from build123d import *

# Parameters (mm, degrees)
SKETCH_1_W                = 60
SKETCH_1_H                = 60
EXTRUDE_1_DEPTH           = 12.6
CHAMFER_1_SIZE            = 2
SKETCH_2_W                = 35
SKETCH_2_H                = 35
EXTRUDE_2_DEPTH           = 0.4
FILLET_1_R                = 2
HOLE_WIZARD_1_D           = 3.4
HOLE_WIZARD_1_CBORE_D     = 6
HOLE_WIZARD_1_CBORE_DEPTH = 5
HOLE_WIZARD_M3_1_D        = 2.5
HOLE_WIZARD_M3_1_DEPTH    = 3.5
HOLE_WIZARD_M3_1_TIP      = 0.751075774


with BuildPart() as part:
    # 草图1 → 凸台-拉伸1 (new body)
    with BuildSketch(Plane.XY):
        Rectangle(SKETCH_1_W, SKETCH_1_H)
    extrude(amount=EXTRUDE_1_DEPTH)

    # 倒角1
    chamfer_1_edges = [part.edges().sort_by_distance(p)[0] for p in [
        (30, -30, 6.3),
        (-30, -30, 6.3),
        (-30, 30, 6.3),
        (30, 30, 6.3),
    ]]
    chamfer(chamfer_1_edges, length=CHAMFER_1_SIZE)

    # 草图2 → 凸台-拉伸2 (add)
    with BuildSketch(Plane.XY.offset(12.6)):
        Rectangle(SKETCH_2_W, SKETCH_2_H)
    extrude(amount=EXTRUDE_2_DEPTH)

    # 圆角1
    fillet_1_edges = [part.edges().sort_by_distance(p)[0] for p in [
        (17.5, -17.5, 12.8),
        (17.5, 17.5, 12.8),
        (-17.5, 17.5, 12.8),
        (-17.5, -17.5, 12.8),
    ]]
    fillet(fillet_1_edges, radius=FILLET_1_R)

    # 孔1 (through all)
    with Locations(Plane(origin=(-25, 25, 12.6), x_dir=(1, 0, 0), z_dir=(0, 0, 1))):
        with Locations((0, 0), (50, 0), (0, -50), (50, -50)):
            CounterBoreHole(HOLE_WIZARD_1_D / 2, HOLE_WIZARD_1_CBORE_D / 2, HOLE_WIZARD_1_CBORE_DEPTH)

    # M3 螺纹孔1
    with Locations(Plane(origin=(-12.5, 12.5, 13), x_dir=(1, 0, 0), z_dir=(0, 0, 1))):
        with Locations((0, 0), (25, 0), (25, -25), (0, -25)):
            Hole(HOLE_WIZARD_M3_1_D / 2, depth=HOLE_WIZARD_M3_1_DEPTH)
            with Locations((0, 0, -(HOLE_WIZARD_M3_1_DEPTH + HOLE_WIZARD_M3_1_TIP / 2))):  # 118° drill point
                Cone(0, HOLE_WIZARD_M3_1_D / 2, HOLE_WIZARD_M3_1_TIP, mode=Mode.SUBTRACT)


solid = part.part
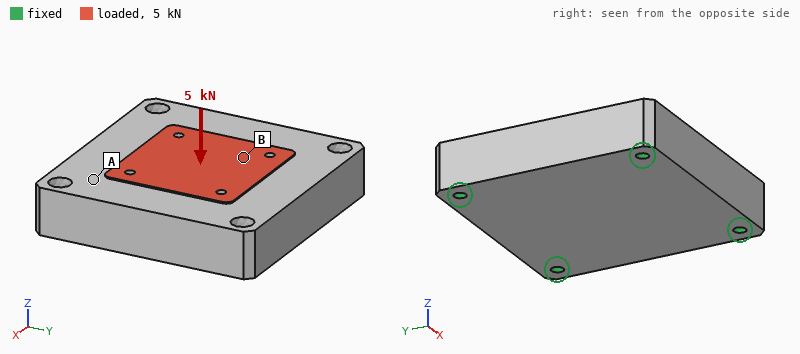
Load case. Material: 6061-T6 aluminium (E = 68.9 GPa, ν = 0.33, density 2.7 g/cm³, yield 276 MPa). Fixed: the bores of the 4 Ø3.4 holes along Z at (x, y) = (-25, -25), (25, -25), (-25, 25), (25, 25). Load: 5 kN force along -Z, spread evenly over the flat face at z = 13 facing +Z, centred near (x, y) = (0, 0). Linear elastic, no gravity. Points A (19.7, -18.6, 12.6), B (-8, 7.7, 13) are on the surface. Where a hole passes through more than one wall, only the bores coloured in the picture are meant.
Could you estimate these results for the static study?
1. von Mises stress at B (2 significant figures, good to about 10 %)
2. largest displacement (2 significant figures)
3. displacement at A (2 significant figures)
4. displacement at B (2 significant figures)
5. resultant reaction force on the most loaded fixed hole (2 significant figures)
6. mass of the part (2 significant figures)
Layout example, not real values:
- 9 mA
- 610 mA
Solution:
- 15 MPa
- 18 µm
- 7.7 µm
- 16 µm
- 1.5 kN
- 120 g
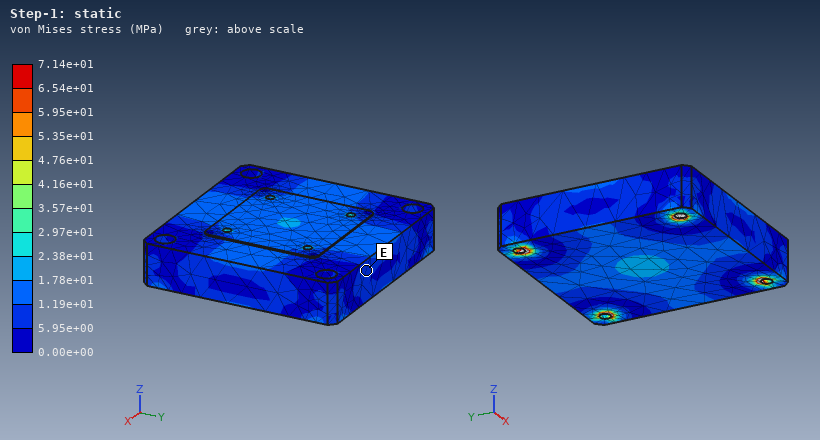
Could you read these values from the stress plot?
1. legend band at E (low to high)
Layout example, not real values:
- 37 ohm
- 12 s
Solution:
- 5.95e+00 to 1.19e+01 MPa
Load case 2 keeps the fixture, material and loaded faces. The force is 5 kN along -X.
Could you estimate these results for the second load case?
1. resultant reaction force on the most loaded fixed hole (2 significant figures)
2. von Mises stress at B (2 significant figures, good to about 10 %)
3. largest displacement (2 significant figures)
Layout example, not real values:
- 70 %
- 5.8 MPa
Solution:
- 1.4 kN
- 8.5 MPa
- 5.6 µm
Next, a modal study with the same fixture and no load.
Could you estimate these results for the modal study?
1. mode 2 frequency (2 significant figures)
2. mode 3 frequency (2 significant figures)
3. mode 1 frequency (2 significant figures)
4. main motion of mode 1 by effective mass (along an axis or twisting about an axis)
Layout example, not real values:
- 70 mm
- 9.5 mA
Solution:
- 17 kHz
- 17 kHz
- 11 kHz
- along Z
